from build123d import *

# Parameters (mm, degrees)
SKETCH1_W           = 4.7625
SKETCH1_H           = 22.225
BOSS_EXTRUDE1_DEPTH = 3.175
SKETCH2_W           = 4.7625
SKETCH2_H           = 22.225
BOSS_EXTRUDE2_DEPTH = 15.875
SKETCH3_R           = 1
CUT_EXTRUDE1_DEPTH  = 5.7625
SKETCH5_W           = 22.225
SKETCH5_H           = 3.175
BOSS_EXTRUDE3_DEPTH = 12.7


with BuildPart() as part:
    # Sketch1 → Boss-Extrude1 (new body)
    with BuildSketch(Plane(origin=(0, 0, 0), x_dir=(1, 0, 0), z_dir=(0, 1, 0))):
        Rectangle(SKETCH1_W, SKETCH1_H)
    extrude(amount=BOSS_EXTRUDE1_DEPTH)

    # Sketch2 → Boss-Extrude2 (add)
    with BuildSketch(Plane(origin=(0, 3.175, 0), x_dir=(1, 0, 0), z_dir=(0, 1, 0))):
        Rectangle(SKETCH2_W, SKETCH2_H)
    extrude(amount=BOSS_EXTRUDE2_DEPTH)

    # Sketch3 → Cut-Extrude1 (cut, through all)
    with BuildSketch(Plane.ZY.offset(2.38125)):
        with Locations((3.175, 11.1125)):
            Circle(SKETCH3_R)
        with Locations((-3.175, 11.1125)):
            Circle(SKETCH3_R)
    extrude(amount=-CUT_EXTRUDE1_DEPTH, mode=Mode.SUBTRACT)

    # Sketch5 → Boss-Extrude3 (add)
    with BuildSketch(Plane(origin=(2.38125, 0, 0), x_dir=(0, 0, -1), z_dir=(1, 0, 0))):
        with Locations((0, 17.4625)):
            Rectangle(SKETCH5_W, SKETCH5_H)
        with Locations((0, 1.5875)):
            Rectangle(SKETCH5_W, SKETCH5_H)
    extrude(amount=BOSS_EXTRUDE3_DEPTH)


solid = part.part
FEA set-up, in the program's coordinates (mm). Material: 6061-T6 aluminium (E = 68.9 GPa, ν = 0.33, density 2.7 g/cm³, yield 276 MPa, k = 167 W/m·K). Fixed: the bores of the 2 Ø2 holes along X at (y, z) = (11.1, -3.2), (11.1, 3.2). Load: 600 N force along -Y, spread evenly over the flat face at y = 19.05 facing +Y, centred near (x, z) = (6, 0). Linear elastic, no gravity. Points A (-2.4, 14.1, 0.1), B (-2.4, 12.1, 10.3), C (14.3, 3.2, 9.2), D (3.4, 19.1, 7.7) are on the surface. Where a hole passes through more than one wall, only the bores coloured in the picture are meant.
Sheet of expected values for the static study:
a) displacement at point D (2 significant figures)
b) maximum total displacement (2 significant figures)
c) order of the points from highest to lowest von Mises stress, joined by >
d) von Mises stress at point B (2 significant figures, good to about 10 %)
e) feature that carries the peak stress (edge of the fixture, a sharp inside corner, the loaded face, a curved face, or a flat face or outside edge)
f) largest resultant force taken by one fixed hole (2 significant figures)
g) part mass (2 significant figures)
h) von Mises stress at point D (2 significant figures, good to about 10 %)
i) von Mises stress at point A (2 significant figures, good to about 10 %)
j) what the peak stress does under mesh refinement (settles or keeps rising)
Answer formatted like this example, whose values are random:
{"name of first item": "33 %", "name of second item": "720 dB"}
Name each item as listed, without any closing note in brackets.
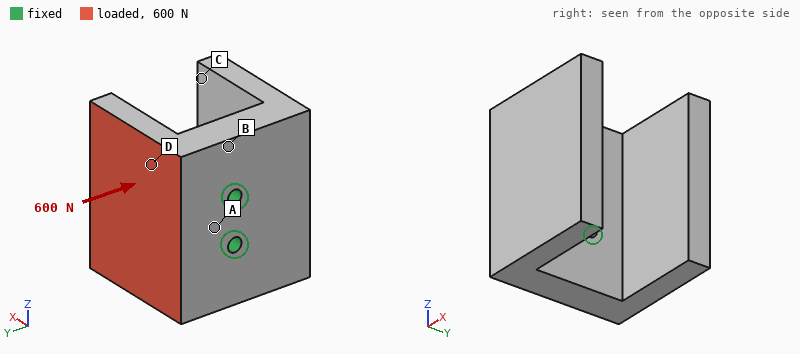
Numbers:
{"displacement at point D": "16 µm", "maximum total displacement": "69 µm", "order of the points from highest to lowest von Mises stress, joined by >": "D > A > B > C", "von Mises stress at point B": "24 MPa", "feature that carries the peak stress": "edge of the fixture", "largest resultant force taken by one fixed hole": "300 N", "part mass": "10 g", "von Mises stress at point D": "53 MPa", "von Mises stress at point A": "38 MPa", "what the peak stress does under mesh refinement": "keeps rising"}
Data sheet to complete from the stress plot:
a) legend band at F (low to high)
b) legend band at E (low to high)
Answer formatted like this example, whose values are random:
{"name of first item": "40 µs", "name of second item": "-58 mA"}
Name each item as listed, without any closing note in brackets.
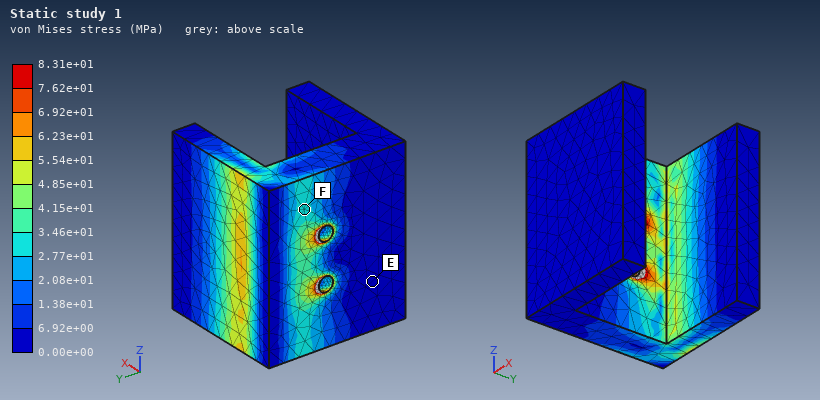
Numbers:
{"legend band at F": "2.77e+01 to 3.46e+01 MPa", "legend band at E": "0.00e+00 to 6.92e+00 MPa"}
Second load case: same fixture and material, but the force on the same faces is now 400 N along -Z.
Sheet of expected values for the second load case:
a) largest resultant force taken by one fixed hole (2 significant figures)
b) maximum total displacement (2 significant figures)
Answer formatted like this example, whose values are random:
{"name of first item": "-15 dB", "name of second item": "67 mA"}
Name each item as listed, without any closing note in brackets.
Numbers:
{"largest resultant force taken by one fixed hole": "490 N", "maximum total displacement": "14 µm"}
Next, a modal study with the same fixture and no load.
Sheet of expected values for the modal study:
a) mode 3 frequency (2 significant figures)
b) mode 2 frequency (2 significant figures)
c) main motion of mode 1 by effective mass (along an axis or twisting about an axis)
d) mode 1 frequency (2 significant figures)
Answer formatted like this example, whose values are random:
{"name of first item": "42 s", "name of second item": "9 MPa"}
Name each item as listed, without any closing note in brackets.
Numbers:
{"mode 3 frequency": "12 kHz", "mode 2 frequency": "10 kHz", "main motion of mode 1 by effective mass": "along Y", "mode 1 frequency": "8300 Hz"}
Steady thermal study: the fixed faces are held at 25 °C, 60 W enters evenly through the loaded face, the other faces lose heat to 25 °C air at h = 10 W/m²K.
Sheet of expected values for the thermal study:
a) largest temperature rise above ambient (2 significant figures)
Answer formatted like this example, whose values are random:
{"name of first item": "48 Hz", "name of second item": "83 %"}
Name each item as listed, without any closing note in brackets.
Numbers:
{"largest temperature rise above ambient": "53 K"}
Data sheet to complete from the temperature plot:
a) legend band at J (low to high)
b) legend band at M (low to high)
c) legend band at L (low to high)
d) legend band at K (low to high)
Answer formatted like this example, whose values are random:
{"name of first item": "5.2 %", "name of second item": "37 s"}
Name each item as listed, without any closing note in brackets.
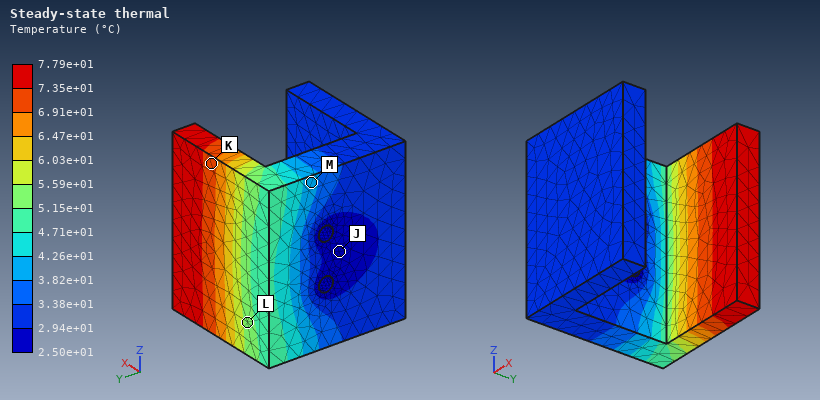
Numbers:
{"legend band at J": "2.50e+01 to 2.94e+01 °C", "legend band at M": "3.82e+01 to 4.26e+01 °C", "legend band at L": "5.15e+01 to 5.59e+01 °C", "legend band at K": "6.91e+01 to 7.35e+01 °C"}
